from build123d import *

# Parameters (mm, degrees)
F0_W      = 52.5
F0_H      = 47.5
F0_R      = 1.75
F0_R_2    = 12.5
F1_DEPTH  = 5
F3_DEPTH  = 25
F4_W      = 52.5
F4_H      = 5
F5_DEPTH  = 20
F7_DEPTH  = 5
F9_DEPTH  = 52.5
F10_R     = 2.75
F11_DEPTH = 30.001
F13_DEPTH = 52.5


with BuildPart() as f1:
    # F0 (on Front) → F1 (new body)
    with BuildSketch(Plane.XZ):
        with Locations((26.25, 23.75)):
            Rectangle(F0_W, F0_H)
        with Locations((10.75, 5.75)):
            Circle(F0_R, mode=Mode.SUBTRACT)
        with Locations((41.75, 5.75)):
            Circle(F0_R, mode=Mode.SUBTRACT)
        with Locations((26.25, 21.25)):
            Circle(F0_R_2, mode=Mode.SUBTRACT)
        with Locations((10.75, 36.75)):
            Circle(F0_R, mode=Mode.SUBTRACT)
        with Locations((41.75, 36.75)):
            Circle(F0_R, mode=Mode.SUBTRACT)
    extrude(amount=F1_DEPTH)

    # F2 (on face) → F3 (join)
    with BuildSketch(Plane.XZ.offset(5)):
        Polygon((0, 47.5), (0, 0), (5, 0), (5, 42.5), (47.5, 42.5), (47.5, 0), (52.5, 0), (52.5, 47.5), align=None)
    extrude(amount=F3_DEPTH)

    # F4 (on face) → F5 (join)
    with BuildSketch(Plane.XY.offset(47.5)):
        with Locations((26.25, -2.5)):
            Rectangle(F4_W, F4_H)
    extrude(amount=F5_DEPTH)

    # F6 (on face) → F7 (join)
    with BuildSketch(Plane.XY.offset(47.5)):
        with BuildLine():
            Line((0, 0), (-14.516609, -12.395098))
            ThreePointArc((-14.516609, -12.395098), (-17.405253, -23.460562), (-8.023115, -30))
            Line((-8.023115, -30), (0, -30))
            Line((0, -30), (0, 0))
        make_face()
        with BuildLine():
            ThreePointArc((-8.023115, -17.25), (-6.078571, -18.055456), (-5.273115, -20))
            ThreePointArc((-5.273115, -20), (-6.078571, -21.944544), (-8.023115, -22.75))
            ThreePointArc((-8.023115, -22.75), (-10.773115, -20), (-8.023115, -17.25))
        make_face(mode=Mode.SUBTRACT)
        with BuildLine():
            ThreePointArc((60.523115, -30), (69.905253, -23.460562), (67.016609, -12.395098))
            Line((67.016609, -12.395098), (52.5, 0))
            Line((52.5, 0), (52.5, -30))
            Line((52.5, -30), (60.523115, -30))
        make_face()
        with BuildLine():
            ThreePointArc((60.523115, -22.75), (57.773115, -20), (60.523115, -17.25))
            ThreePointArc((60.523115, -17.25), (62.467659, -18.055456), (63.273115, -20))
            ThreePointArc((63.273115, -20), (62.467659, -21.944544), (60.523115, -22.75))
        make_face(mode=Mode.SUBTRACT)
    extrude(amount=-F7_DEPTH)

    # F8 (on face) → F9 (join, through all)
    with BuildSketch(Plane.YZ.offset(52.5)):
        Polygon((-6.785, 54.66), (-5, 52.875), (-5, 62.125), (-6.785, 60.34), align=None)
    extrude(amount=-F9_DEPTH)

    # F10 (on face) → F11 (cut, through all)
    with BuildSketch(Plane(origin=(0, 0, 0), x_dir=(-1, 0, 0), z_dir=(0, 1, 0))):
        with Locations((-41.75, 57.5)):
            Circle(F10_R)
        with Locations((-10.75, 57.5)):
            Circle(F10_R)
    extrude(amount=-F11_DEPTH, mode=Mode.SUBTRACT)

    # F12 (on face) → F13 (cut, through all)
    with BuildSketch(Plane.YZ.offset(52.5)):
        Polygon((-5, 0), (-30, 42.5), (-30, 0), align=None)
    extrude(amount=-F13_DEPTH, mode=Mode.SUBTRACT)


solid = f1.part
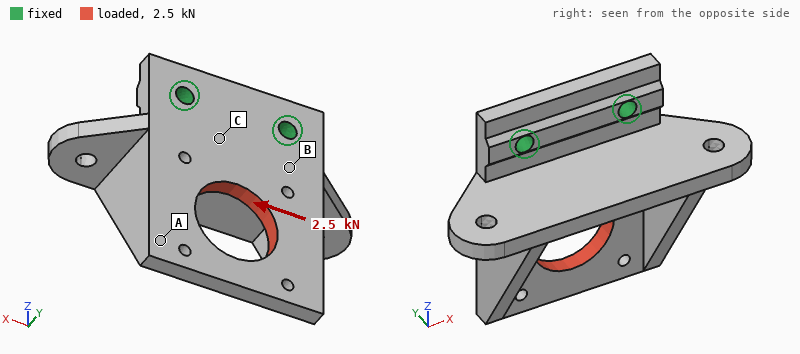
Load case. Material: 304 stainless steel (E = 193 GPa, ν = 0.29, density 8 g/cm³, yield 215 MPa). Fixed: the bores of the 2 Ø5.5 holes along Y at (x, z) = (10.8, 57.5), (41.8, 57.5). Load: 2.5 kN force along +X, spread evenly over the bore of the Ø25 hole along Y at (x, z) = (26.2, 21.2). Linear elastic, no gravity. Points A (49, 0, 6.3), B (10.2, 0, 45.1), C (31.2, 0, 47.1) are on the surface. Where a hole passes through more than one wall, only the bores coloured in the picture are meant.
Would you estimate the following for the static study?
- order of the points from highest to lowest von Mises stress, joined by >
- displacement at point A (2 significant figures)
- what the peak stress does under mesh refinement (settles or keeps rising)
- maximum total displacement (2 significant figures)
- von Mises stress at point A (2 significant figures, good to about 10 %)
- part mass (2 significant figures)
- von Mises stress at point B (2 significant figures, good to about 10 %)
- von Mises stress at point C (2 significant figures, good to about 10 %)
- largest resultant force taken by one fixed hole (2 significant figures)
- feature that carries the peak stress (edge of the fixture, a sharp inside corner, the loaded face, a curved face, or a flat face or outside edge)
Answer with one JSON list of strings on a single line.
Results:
["C > B > A", "20 µm", "keeps rising", "23 µm", "8.8 MPa", "250 g", "17 MPa", "33 MPa", "2.8 kN", "edge of the fixture"]
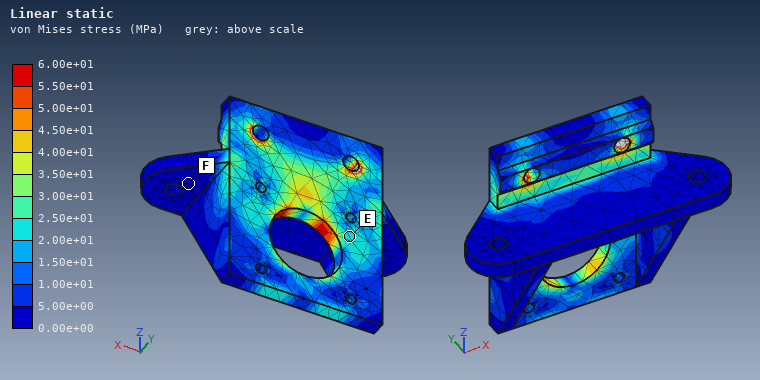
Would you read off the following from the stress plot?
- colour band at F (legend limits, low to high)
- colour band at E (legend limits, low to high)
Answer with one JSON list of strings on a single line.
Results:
["0.00e+00 to 5.00e+00 MPa", "2.00e+01 to 2.50e+01 MPa"]
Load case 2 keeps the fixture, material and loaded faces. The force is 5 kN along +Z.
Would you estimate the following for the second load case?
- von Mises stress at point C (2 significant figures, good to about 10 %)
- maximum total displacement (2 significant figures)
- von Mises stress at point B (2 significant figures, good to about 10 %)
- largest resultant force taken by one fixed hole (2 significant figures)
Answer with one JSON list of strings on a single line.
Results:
["15 MPa", "15 µm", "26 MPa", "2.5 kN"]
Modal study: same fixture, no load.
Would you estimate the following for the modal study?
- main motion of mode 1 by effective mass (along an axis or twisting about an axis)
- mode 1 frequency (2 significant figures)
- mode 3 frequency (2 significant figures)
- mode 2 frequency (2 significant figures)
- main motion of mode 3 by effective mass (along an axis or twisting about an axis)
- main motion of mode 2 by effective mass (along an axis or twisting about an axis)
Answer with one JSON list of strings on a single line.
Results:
["along Y", "1300 Hz", "5400 Hz", "2800 Hz", "along X", "twisting about Z"]
